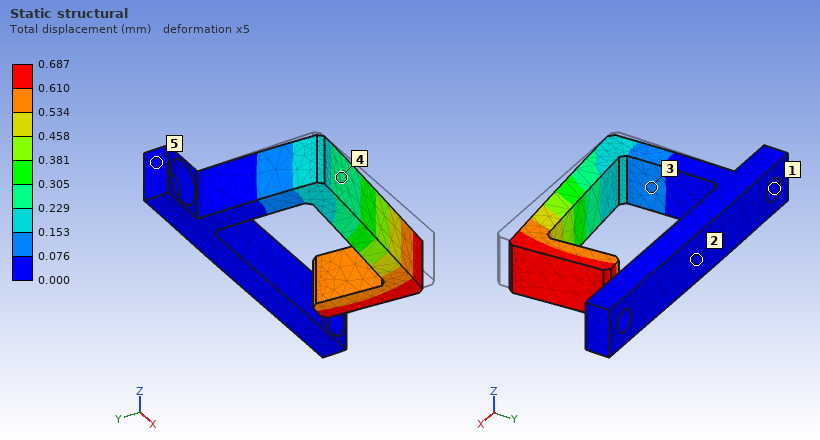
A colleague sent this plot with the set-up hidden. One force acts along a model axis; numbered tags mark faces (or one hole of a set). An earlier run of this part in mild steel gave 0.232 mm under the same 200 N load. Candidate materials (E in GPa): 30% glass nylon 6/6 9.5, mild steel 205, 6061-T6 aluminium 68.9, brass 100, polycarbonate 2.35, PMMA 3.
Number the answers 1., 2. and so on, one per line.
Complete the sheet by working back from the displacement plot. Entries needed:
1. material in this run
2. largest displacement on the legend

1. 6061-T6 aluminium
2. 0.687 mm
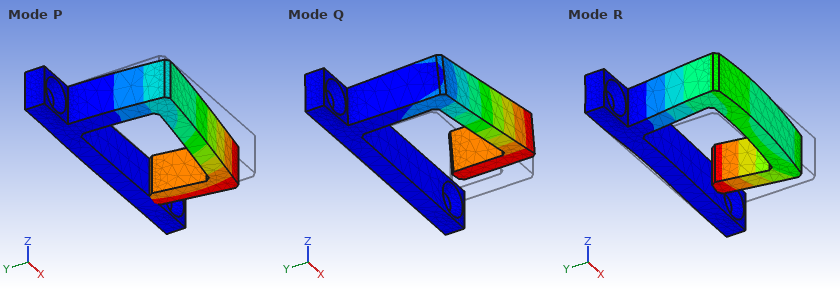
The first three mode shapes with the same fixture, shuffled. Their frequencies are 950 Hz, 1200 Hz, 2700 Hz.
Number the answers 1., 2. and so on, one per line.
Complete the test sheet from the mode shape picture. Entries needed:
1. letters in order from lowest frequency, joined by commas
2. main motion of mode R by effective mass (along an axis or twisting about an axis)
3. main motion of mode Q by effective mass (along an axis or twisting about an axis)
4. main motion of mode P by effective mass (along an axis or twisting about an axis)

1. P, Q, R
2. along X
3. along Z
4. along Y
